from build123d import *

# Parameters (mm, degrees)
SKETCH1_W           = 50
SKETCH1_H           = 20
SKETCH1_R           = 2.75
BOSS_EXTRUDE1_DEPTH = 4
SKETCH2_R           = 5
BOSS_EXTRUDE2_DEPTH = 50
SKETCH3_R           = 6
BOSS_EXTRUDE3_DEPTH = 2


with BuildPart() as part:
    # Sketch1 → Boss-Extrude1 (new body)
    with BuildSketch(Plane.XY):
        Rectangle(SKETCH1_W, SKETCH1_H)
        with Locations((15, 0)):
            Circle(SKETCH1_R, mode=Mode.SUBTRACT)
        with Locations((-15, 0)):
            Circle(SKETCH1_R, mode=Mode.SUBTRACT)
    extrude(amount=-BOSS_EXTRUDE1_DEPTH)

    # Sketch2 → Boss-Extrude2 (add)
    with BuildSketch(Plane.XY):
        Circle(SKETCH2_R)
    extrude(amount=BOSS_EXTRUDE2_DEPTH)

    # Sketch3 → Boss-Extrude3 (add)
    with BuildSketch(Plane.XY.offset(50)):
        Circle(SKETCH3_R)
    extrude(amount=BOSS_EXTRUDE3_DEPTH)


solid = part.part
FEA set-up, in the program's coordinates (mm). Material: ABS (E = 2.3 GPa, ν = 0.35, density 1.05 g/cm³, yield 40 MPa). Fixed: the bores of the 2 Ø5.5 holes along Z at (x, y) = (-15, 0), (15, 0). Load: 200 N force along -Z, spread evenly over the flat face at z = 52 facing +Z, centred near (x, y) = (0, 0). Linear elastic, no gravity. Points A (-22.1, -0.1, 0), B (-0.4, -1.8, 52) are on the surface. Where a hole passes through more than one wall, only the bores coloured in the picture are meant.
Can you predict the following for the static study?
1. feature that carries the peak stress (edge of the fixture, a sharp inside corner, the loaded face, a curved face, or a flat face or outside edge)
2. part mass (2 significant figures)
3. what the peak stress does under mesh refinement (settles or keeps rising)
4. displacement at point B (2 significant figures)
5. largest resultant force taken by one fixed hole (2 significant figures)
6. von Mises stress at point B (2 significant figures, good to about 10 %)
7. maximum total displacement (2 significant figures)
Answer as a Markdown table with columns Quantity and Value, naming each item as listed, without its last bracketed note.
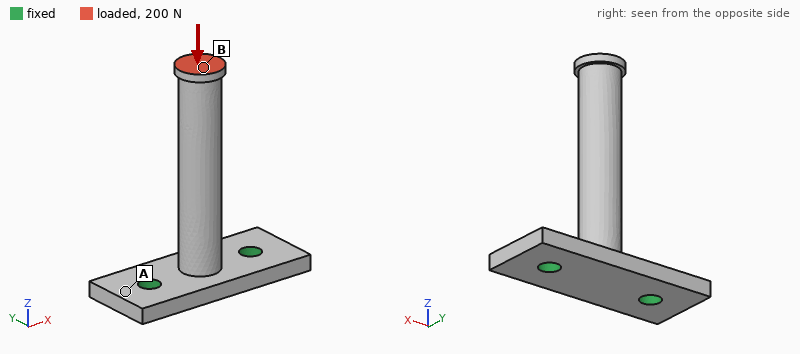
| Quantity | Value |
|---|---|
| feature that carries the peak stress | edge of the fixture |
| part mass | 8.4 g |
| what the peak stress does under mesh refinement | keeps rising |
| displacement at point B | 0.13 mm |
| largest resultant force taken by one fixed hole | 100 N |
| von Mises stress at point B | 3.0 MPa |
| maximum total displacement | 0.14 mm |
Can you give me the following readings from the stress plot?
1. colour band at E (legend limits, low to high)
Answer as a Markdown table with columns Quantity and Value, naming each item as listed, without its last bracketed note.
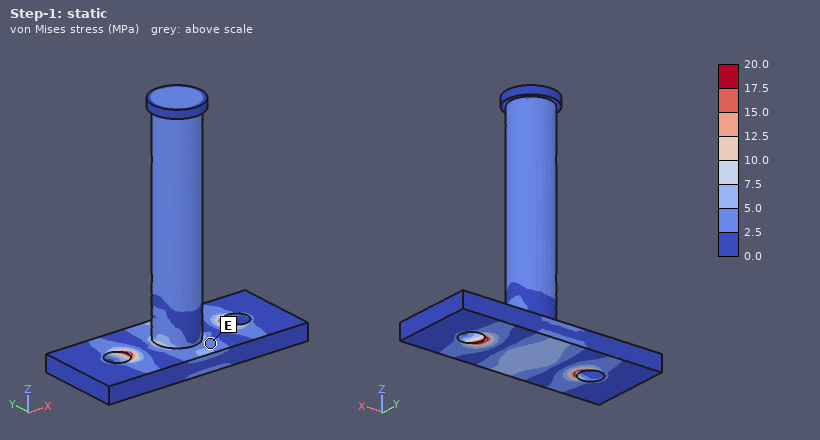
| Quantity | Value |
|---|---|
| colour band at E | 2.5 to 5.0 MPa |
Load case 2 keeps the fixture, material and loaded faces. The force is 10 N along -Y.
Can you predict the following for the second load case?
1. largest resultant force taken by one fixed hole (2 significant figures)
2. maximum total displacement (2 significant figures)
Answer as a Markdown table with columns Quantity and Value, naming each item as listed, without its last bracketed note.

| Quantity | Value |
|---|---|
| largest resultant force taken by one fixed hole | 5.0 N |
| maximum total displacement | 0.84 mm |
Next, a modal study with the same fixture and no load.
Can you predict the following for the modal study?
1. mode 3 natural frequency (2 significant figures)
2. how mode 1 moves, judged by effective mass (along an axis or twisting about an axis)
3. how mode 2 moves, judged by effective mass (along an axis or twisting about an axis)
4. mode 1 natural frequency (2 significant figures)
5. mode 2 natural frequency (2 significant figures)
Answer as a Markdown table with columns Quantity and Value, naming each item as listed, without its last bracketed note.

| Quantity | Value |
|---|---|
| mode 3 natural frequency | 3100 Hz |
| how mode 1 moves, judged by effective mass | along Y |
| how mode 2 moves, judged by effective mass | along X |
| mode 1 natural frequency | 480 Hz |
| mode 2 natural frequency | 600 Hz |
